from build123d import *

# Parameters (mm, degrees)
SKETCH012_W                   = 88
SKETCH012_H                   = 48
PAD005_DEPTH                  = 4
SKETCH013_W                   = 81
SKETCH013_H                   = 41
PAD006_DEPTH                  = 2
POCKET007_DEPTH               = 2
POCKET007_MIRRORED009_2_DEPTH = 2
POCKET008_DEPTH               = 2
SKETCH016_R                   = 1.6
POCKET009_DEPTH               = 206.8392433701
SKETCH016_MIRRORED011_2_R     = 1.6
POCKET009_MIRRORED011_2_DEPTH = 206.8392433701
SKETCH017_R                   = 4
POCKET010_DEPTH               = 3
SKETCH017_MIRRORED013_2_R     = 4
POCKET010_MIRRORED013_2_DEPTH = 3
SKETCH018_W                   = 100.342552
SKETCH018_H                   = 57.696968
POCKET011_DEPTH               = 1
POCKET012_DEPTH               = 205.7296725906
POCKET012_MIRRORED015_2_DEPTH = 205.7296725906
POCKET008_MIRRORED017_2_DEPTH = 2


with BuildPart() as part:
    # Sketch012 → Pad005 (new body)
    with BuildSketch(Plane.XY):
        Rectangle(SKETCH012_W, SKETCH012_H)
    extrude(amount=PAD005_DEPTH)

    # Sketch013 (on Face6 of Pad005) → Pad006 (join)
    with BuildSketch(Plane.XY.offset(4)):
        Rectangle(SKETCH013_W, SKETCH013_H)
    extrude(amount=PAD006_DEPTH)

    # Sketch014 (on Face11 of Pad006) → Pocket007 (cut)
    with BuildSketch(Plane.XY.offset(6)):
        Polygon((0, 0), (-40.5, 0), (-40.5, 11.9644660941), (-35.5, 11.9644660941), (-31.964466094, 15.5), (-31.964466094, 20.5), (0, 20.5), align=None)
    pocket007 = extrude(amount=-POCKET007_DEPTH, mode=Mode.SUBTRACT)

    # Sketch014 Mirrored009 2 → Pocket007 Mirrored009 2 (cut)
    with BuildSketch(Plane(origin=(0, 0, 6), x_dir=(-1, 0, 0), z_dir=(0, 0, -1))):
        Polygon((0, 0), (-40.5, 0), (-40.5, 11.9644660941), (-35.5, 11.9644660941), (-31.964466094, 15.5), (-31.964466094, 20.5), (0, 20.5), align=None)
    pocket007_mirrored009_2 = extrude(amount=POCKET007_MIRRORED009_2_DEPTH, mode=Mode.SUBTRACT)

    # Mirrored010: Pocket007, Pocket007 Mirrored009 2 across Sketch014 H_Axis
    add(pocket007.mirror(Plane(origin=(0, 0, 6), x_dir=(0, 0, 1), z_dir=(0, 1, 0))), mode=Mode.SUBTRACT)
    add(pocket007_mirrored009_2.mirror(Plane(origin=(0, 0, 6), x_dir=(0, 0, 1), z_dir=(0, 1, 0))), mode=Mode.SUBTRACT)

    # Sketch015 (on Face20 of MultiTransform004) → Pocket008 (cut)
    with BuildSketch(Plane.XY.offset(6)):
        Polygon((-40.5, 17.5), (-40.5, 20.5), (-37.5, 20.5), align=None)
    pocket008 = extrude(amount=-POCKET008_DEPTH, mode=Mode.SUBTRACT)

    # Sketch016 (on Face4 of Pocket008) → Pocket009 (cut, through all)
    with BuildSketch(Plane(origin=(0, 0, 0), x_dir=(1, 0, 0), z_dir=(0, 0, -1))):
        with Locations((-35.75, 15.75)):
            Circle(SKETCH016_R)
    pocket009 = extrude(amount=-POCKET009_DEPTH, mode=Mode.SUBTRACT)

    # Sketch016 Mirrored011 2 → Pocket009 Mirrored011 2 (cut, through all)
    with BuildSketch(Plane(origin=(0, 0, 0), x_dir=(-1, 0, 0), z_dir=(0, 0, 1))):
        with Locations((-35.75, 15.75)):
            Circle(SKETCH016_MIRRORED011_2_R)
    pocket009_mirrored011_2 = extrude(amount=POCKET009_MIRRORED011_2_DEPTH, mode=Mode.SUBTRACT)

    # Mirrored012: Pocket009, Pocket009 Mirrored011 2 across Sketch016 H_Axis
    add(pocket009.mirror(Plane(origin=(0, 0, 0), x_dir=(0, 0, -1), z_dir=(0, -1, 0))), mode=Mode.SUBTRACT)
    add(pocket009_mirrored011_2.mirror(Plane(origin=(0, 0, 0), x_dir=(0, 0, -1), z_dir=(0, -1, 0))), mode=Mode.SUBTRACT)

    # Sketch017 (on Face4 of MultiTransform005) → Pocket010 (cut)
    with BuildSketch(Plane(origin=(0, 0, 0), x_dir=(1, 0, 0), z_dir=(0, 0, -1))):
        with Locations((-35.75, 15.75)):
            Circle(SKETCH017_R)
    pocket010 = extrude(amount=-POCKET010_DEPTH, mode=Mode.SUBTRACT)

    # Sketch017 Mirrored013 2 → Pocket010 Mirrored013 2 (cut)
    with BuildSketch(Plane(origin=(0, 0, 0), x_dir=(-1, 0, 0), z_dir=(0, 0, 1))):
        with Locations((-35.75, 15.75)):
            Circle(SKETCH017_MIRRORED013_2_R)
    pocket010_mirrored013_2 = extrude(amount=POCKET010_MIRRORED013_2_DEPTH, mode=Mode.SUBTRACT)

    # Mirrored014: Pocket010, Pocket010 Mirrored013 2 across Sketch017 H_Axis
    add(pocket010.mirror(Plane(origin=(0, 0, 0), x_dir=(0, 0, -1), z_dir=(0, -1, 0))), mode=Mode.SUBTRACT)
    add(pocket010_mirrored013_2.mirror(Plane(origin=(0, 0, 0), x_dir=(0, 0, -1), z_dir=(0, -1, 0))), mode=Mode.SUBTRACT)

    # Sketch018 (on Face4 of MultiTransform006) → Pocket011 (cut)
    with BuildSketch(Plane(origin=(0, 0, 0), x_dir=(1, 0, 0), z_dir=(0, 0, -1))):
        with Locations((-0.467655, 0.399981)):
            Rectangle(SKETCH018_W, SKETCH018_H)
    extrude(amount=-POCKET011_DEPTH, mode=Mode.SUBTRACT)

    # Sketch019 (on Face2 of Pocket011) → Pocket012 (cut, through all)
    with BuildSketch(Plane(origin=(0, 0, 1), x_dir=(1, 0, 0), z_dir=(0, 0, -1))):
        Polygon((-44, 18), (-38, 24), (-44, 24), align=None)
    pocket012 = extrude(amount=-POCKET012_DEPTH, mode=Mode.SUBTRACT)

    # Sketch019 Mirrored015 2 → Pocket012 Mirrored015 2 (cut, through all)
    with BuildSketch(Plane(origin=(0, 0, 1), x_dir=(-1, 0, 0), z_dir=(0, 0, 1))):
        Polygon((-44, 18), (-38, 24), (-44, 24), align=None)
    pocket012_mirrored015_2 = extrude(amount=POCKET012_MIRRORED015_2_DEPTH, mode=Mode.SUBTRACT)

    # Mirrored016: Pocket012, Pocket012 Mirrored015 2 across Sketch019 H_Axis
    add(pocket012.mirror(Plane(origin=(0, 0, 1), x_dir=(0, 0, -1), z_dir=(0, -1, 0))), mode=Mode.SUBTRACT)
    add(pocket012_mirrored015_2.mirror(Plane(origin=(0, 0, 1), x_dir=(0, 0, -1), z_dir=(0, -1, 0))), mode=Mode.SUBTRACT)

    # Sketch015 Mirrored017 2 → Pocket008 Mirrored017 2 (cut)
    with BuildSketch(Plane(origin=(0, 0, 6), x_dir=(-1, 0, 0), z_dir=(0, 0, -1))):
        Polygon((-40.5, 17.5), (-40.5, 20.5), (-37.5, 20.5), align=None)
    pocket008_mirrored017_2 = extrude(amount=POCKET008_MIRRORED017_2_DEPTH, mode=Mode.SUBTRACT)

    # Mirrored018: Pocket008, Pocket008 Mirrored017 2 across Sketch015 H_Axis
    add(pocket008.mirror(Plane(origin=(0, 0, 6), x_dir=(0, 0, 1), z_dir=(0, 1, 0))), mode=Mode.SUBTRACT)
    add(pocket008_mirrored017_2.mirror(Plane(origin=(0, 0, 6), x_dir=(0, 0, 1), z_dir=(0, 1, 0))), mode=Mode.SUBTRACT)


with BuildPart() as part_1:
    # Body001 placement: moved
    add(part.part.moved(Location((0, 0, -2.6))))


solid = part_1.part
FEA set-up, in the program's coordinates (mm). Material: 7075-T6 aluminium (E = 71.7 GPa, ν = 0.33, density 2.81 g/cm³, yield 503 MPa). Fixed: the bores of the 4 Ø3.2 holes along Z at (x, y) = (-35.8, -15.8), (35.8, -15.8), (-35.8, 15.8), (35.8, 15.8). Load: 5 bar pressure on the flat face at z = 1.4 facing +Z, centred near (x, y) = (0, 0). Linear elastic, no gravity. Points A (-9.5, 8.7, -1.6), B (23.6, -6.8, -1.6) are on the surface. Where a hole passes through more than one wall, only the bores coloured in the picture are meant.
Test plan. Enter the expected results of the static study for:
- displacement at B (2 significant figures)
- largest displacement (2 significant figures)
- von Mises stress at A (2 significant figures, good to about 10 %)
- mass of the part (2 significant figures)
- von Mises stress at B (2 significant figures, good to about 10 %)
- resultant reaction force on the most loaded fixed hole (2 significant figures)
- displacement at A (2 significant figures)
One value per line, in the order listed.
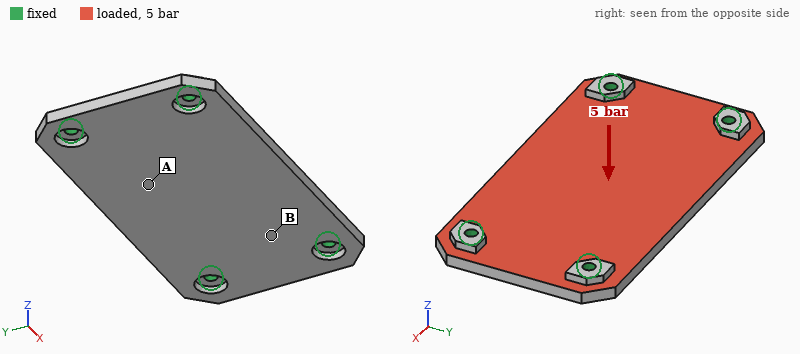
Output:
0.11 mm
0.27 mm
69 MPa
35 g
25 MPa
970 N
0.23 mm
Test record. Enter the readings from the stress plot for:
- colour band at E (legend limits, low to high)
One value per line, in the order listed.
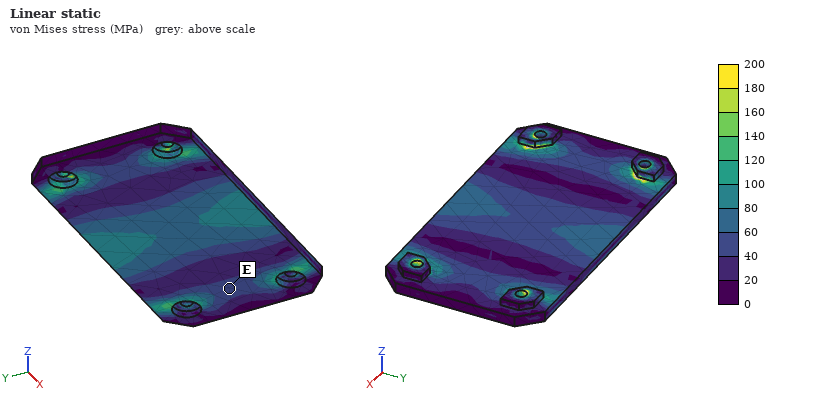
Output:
40 to 60 MPa
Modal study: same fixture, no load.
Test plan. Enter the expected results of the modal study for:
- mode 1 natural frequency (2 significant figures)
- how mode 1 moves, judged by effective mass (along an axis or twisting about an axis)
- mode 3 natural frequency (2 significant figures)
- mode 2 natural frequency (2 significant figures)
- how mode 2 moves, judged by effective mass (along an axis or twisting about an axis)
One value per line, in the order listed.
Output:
2700 Hz
along Z
7100 Hz
4100 Hz
twisting about X
